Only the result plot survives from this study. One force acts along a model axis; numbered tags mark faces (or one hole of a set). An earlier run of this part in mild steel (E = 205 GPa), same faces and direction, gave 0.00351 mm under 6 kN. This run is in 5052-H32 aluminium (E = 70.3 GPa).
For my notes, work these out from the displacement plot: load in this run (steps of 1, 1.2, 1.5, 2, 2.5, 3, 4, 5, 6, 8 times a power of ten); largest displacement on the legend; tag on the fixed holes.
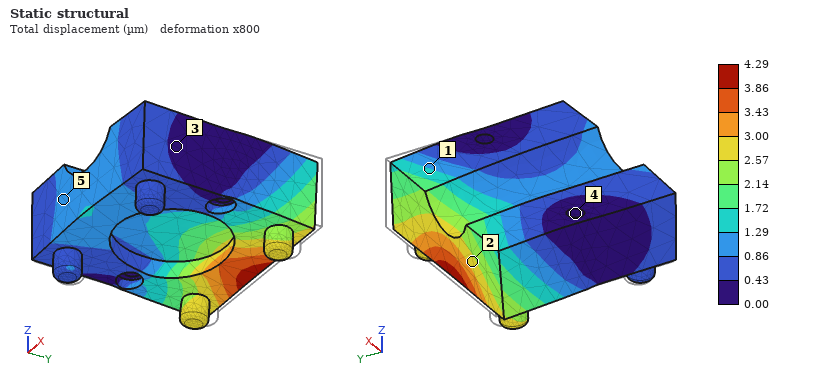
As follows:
2.5 kN
4.29 µm
4
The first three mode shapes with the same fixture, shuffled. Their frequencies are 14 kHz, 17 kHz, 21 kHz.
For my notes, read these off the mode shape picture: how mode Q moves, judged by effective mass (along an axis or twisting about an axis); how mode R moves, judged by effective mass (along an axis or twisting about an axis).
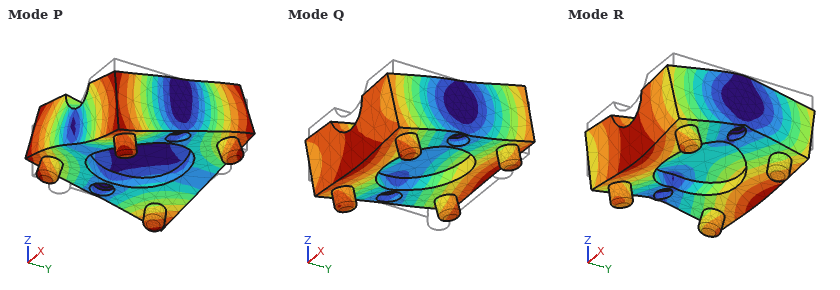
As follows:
twisting about X
along Z
